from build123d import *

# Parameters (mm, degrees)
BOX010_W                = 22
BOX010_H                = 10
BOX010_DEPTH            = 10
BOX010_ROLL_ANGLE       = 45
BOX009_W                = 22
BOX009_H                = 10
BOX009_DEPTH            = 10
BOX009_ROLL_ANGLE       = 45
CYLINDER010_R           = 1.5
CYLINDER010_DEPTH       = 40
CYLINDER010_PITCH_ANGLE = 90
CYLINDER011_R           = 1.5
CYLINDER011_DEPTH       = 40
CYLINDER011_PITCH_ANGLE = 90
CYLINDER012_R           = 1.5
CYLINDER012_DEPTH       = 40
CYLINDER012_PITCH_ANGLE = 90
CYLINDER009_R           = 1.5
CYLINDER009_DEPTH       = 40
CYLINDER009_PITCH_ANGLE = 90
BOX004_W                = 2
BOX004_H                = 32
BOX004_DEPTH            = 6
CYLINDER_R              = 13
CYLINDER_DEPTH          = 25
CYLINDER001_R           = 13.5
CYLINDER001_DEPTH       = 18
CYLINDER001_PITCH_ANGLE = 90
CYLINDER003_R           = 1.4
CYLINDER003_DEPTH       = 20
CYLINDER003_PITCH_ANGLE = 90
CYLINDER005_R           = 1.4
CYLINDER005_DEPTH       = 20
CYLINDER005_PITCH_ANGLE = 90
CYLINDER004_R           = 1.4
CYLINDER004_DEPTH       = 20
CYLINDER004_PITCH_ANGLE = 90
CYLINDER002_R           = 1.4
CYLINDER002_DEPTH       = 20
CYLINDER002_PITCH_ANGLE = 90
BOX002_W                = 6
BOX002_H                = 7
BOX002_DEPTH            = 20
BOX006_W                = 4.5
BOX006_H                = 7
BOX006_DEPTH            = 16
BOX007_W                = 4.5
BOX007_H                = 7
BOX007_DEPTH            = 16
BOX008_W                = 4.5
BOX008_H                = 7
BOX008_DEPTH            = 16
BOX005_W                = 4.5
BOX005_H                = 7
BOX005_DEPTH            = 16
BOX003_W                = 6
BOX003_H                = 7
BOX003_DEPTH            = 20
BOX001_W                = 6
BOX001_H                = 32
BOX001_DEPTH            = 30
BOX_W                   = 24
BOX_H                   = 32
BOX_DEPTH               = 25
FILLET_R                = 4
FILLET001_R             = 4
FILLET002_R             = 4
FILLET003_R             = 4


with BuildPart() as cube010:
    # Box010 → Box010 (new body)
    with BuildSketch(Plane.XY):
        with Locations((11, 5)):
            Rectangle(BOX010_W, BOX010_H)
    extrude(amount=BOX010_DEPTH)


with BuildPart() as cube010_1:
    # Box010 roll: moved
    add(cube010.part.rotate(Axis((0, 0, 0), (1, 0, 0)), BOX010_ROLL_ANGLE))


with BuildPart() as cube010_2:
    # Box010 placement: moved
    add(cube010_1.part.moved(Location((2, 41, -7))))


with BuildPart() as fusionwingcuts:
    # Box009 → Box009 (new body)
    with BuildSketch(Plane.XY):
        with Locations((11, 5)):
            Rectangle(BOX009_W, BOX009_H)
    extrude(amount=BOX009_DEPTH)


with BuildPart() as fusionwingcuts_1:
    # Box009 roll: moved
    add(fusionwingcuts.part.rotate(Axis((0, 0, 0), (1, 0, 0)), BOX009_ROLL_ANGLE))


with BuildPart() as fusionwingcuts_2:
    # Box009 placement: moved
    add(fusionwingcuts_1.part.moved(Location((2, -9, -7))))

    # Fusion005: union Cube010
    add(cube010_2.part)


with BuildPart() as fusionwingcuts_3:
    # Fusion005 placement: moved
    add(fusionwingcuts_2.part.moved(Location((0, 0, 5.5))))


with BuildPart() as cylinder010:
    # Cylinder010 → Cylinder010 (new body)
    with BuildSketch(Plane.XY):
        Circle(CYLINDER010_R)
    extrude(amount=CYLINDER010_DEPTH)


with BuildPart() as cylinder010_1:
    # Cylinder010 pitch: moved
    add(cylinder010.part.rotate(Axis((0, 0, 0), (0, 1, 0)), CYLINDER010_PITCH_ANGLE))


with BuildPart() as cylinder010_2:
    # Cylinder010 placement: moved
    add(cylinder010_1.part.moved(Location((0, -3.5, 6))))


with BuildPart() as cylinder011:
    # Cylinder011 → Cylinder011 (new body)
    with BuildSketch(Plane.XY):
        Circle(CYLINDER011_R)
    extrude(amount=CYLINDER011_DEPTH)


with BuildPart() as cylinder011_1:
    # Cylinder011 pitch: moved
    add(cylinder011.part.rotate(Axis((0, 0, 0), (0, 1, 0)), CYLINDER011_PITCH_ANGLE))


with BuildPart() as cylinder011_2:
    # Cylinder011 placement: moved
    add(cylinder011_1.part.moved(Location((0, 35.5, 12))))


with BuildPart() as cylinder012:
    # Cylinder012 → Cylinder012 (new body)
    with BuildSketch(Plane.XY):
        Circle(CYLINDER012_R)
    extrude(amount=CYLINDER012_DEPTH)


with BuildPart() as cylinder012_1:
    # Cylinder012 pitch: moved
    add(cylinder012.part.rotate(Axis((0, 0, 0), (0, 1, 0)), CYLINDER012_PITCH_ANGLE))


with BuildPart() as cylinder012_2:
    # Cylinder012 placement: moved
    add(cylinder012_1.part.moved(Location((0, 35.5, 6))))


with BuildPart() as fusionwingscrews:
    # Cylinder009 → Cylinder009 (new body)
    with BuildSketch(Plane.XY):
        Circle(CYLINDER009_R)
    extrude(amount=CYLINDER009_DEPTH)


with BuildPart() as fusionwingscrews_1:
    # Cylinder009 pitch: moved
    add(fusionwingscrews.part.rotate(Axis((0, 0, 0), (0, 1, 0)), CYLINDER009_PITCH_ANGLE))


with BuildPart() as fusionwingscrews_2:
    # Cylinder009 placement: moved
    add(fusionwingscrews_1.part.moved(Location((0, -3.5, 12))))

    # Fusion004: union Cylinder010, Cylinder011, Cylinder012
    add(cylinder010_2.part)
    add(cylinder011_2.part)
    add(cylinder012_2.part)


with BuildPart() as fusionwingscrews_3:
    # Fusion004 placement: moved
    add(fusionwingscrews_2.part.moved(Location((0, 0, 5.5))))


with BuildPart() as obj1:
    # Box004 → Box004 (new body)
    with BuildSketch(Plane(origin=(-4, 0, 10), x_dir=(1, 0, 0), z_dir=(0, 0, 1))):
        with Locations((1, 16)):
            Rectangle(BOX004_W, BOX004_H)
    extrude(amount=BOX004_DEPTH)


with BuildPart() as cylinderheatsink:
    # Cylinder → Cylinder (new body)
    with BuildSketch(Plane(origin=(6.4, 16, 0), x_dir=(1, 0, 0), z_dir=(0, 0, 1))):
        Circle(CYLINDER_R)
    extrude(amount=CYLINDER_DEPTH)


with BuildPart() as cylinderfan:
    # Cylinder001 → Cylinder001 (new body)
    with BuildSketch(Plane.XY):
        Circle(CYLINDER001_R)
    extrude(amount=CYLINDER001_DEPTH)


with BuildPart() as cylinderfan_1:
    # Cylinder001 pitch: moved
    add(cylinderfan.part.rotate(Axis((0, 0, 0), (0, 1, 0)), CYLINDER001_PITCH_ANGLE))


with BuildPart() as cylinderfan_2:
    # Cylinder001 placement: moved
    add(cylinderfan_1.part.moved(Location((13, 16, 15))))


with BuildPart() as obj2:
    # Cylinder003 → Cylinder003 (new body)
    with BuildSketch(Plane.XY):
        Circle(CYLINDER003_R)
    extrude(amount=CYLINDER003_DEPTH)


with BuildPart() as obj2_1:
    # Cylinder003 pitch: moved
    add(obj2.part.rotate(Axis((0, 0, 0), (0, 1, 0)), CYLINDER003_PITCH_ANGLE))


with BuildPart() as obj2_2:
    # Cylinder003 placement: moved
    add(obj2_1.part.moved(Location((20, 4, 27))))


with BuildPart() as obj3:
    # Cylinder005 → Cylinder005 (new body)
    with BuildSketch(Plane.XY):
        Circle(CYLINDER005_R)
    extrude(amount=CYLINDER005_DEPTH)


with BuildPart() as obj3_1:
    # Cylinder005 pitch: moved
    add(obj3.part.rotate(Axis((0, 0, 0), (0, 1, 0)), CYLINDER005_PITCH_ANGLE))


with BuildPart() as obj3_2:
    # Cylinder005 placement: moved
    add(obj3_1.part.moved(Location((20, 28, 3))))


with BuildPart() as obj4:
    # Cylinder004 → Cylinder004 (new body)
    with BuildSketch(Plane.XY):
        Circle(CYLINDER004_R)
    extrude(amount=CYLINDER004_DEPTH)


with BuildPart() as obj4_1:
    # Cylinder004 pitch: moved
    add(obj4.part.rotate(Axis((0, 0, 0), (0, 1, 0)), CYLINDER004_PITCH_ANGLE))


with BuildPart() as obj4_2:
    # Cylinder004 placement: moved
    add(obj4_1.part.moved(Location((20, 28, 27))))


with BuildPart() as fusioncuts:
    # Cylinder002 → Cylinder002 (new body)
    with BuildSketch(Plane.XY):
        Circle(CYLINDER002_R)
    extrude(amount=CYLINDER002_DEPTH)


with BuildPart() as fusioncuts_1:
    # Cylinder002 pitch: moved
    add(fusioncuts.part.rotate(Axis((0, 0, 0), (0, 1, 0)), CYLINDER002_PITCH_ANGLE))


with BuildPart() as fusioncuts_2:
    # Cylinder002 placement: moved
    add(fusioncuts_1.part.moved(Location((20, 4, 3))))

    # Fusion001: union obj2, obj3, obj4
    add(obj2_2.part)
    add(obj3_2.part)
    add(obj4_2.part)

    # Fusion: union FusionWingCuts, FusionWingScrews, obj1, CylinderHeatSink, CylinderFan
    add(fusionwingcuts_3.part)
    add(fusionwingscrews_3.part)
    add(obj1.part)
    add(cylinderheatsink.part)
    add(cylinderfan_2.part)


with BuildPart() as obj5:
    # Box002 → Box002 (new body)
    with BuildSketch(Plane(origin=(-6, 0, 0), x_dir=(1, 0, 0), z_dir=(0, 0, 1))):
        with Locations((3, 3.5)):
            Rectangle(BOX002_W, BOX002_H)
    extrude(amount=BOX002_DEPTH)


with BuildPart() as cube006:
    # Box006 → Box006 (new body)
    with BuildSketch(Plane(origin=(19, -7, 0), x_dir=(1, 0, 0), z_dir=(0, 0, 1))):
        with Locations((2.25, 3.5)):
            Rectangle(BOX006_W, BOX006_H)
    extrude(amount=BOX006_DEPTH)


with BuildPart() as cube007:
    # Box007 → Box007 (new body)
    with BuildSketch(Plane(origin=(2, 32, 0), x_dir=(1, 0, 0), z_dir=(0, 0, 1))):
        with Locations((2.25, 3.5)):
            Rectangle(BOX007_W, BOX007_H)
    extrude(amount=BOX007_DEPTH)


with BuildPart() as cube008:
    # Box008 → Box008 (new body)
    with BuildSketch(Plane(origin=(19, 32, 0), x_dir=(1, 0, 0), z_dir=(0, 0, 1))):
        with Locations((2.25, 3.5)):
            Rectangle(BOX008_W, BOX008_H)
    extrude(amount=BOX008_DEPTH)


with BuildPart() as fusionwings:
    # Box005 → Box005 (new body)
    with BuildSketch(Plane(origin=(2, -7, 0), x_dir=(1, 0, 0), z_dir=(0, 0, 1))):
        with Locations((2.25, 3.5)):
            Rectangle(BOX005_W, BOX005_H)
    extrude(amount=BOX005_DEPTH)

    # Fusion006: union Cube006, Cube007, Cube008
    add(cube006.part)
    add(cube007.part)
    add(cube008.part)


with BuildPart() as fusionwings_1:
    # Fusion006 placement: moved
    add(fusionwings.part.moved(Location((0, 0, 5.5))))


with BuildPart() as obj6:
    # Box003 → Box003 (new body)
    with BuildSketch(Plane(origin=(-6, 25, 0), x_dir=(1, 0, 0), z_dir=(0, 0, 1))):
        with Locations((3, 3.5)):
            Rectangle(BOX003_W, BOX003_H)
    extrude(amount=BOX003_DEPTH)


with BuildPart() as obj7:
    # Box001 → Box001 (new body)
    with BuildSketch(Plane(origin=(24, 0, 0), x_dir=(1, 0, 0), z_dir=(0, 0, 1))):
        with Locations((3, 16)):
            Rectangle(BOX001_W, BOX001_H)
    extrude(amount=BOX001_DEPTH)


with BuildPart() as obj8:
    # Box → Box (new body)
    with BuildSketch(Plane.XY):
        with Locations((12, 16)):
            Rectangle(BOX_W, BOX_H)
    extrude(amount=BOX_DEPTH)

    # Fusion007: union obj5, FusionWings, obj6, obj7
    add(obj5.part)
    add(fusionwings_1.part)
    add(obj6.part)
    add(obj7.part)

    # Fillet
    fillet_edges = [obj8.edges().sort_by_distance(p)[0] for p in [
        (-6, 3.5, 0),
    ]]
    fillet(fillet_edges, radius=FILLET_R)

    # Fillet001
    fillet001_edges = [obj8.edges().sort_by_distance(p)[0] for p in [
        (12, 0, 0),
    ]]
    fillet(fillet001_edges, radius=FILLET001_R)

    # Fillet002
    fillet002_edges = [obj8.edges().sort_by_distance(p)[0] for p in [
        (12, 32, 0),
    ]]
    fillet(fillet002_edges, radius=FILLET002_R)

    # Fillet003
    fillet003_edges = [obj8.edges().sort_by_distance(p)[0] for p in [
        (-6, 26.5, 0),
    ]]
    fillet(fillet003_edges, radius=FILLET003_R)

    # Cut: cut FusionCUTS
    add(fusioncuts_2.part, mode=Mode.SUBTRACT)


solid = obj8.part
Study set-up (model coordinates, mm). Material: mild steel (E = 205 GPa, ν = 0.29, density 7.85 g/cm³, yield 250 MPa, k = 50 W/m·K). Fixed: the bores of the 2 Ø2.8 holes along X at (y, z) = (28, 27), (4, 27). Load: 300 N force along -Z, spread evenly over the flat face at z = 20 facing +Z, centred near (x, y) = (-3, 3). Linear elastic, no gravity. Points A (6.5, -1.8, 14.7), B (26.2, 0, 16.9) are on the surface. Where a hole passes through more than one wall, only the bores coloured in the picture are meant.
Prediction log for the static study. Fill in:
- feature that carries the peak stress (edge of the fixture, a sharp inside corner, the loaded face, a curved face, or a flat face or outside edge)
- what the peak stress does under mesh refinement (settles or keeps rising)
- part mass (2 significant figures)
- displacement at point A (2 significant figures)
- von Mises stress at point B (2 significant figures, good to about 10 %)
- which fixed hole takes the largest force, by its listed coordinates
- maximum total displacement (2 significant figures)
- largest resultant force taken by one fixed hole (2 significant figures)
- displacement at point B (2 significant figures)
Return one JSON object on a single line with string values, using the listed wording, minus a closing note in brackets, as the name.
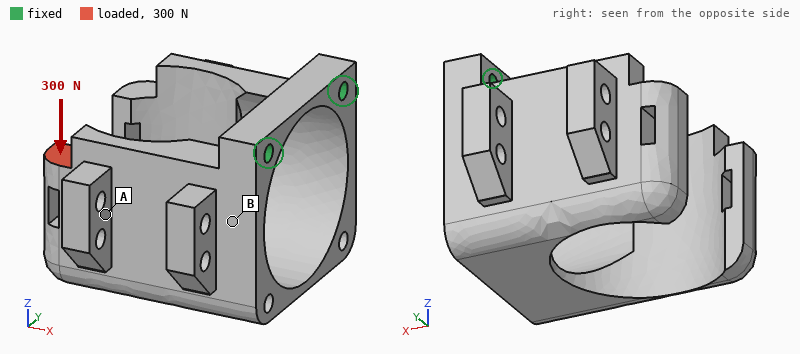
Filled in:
{"feature that carries the peak stress": "a sharp inside corner", "what the peak stress does under mesh refinement": "keeps rising", "part mass": "76 g", "displacement at point A": "41 µm", "von Mises stress at point B": "59 MPa", "which fixed hole takes the largest force, by its listed coordinates": "(4, 27)", "maximum total displacement": "78 µm", "largest resultant force taken by one fixed hole": "290 N", "displacement at point B": "13 µm"}
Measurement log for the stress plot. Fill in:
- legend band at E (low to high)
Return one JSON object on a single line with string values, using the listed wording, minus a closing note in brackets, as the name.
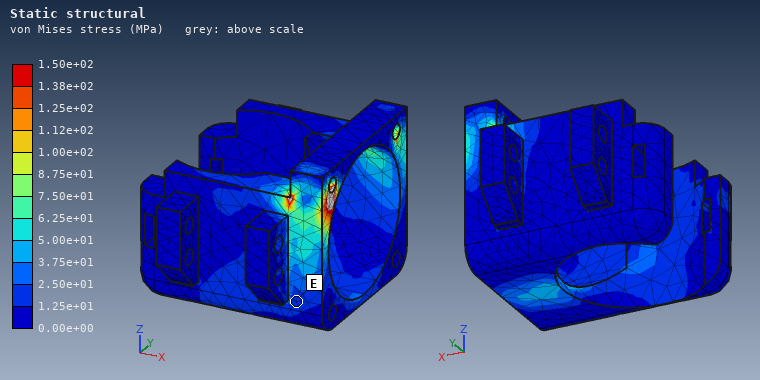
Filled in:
{"legend band at E": "1.25e+01 to 2.50e+01 MPa"}
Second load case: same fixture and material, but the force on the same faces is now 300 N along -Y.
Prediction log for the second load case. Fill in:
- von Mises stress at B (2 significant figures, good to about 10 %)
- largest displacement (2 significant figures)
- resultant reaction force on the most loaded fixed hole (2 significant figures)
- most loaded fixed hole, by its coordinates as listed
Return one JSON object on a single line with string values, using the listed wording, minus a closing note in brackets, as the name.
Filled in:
{"von Mises stress at B": "48 MPa", "largest displacement": "0.13 mm", "resultant reaction force on the most loaded fixed hole": "310 N", "most loaded fixed hole, by its coordinates as listed": "(4, 27)"}
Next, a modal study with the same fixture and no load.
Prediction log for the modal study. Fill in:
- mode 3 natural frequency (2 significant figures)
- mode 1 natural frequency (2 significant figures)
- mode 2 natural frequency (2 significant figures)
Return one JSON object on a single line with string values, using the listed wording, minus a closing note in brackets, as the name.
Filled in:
{"mode 3 natural frequency": "3200 Hz", "mode 1 natural frequency": "2200 Hz", "mode 2 natural frequency": "2300 Hz"}
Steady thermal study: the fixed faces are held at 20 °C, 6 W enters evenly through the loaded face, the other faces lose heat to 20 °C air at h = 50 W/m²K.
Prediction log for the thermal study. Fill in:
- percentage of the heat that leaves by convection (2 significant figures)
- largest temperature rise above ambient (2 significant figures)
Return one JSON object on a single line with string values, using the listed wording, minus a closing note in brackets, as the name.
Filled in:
{"percentage of the heat that leaves by convection": "56 %", "largest temperature rise above ambient": "53 K"}
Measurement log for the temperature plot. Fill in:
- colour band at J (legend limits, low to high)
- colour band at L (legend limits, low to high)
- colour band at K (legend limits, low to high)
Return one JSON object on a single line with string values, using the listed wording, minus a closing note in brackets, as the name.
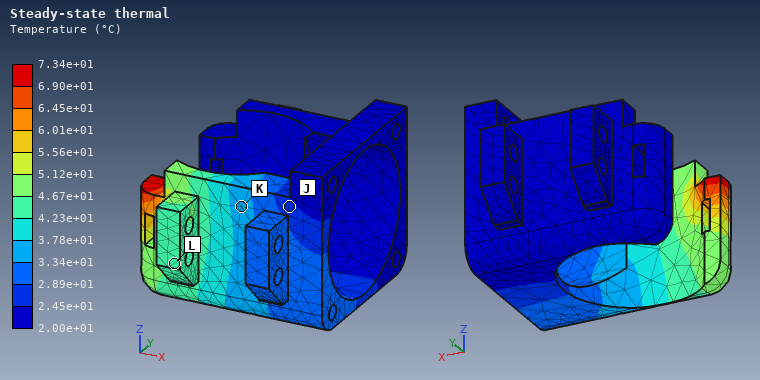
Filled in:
{"colour band at J": "2.45e+01 to 2.89e+01 °C", "colour band at L": "4.23e+01 to 4.67e+01 °C", "colour band at K": "3.34e+01 to 3.78e+01 °C"}
